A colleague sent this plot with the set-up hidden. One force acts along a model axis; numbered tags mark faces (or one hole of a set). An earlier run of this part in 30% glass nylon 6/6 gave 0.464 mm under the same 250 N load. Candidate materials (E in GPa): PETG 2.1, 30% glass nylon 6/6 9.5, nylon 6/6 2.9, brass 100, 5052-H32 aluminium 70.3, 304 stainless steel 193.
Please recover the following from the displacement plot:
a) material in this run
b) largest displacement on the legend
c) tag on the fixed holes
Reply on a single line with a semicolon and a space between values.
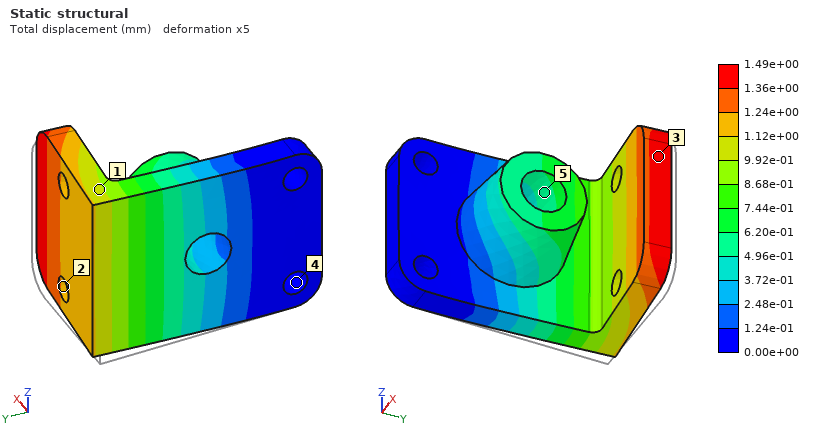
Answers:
nylon 6/6; 1.49e+00 mm; 4
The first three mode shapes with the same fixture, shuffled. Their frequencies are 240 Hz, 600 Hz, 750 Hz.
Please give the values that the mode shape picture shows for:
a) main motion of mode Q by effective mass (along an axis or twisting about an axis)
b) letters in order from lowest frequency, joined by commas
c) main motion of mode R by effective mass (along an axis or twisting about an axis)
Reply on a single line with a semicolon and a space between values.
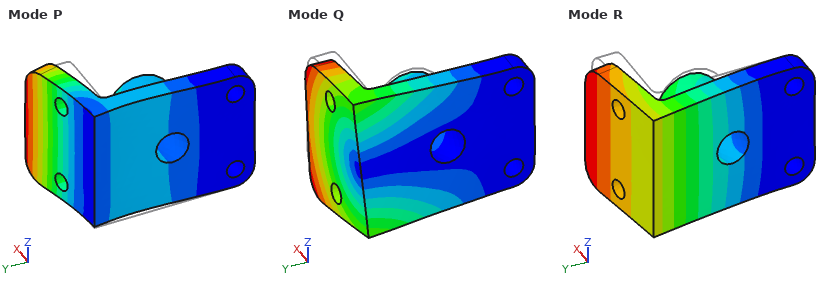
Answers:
along Z; R, Q, P; along X
